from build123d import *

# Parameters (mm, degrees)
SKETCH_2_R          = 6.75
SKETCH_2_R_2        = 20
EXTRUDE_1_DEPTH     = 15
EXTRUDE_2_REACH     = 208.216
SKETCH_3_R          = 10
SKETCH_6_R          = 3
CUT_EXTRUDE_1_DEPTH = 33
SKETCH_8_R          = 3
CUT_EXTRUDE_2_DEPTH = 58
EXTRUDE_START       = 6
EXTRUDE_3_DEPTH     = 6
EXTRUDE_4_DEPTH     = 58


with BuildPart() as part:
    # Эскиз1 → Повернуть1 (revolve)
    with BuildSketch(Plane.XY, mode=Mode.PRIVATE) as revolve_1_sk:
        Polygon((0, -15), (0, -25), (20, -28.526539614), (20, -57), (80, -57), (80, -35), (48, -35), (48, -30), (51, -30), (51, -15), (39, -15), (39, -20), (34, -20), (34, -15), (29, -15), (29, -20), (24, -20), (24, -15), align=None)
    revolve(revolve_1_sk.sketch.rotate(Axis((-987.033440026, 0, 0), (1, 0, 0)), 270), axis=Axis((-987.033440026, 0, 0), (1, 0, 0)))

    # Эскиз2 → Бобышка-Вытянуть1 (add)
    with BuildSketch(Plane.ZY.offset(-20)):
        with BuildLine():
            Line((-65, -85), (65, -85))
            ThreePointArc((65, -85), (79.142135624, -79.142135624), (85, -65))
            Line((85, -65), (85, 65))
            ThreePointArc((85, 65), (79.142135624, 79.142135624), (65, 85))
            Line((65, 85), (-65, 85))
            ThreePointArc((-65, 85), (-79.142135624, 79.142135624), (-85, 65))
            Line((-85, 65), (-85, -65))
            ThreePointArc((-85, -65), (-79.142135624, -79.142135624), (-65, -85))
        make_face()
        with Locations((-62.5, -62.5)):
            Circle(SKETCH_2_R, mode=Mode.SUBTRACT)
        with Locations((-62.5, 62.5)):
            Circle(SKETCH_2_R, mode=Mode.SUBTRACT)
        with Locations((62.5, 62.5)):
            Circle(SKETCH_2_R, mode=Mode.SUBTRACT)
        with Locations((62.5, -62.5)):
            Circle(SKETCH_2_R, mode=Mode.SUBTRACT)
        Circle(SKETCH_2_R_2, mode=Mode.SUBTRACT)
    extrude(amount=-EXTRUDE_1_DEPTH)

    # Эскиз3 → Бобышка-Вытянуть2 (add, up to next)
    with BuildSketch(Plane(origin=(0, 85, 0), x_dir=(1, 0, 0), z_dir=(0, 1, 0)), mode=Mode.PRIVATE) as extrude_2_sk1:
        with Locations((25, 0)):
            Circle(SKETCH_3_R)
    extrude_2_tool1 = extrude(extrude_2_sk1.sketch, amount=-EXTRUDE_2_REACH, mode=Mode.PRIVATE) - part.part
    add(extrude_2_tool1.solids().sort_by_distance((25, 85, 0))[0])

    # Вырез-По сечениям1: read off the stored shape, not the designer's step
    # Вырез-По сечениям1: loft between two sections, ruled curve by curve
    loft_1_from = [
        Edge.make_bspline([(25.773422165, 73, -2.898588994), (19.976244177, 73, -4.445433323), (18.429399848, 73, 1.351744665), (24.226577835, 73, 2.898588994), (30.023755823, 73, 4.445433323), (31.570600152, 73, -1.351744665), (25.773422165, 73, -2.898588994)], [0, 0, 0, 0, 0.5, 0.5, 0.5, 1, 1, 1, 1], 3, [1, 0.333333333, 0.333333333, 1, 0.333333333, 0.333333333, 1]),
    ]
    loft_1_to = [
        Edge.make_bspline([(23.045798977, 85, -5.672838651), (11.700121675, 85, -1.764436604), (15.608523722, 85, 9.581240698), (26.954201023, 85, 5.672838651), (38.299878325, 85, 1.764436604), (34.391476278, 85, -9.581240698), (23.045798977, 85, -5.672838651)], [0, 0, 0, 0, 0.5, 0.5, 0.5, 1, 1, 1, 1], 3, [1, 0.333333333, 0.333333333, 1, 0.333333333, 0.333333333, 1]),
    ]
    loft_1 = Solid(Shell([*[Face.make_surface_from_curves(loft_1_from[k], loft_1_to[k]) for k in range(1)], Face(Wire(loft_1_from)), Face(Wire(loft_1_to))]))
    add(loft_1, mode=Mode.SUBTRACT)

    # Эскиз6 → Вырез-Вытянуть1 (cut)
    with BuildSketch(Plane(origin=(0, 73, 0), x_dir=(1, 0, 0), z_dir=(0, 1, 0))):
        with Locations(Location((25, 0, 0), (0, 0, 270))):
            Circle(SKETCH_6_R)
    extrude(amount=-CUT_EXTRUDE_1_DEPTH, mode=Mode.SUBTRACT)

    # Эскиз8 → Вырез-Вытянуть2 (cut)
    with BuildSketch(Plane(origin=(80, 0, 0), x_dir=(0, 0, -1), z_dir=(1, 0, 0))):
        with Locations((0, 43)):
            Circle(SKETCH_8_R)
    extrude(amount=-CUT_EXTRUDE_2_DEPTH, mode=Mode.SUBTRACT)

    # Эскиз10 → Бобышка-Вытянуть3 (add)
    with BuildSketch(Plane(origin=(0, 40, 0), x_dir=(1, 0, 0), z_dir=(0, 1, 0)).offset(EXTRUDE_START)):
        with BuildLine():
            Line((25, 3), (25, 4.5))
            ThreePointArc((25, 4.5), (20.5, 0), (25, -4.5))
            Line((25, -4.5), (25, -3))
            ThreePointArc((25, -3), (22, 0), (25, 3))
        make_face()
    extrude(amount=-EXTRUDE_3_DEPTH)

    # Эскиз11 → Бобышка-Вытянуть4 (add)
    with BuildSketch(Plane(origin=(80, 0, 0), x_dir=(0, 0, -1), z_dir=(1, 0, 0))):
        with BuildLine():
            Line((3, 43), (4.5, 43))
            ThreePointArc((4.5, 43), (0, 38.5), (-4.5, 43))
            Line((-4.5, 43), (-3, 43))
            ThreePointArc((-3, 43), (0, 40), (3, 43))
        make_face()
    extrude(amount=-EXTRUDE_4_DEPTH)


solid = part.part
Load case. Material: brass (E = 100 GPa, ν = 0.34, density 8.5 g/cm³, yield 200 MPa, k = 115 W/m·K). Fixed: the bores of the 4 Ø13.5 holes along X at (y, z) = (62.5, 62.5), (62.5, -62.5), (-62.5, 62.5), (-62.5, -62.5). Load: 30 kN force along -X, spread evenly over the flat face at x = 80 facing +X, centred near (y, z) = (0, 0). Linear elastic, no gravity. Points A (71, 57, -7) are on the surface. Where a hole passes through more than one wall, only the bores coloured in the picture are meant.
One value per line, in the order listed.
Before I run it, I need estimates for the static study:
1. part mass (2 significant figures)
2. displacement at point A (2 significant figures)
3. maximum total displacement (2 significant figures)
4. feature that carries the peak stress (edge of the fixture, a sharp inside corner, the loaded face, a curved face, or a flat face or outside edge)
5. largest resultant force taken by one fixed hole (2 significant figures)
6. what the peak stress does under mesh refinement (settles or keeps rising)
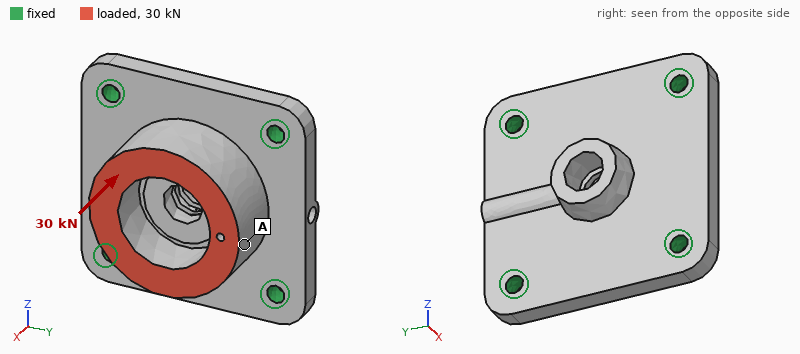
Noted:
6.5 kg
32 µm
34 µm
edge of the fixture
7.9 kN
keeps rising
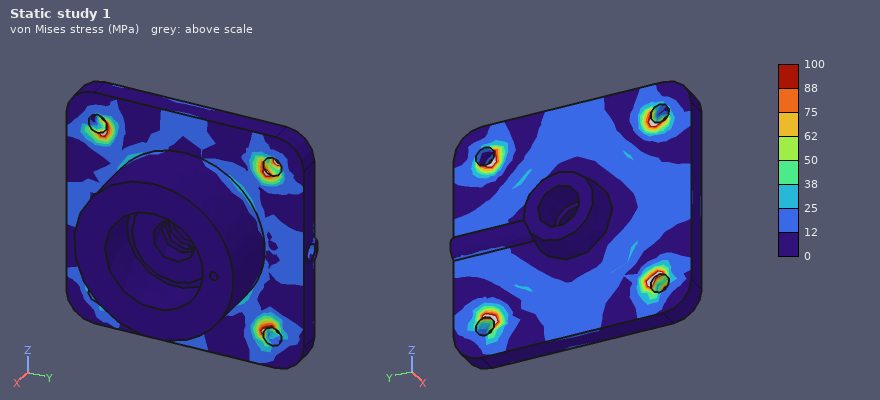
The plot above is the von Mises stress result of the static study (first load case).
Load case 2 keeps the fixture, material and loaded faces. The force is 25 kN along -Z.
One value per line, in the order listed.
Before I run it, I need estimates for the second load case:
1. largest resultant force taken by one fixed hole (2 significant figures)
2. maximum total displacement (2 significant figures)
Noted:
9.0 kN
51 µm
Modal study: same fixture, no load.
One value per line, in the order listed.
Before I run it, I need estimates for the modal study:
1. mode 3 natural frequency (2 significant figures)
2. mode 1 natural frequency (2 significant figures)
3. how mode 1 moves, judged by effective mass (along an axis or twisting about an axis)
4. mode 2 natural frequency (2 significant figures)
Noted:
2700 Hz
2200 Hz
along X
2700 Hz
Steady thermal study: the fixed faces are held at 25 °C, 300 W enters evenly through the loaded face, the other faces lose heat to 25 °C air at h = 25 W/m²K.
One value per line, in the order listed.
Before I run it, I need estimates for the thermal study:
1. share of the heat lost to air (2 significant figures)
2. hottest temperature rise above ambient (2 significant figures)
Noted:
16 %
41 K
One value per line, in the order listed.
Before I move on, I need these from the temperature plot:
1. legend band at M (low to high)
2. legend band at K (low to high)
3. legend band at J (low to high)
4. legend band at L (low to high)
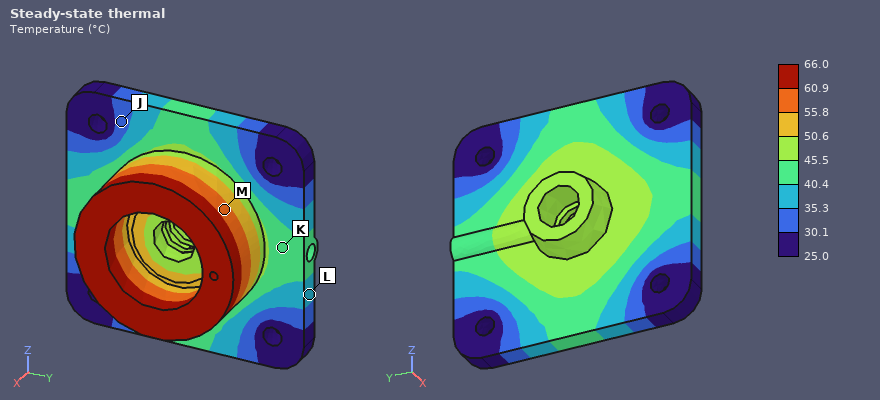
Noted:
55.8 to 60.9 °C
40.4 to 45.5 °C
30.1 to 35.3 °C
35.3 to 40.4 °C
